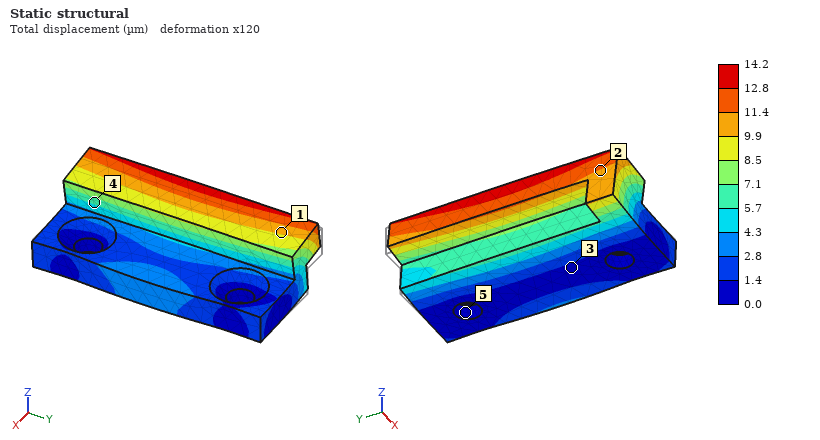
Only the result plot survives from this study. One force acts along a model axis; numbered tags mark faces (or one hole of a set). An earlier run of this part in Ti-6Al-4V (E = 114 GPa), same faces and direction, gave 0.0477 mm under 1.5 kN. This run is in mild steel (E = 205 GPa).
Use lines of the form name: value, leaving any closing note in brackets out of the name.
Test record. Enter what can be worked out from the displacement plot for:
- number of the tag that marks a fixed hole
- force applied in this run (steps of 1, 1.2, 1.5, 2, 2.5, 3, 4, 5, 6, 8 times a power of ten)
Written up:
number of the tag that marks a fixed hole: 5
force applied in this run: 800 N
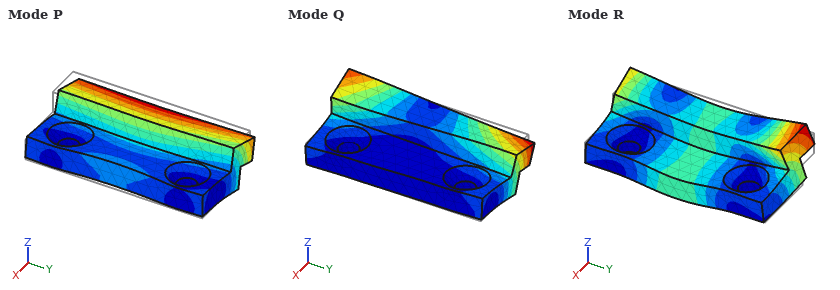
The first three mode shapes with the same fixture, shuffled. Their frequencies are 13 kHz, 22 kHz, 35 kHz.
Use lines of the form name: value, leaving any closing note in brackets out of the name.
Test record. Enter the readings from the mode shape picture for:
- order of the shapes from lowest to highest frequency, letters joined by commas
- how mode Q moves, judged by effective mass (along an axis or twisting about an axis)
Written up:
order of the shapes from lowest to highest frequency, letters joined by commas: P, Q, R
how mode Q moves, judged by effective mass: twisting about X
